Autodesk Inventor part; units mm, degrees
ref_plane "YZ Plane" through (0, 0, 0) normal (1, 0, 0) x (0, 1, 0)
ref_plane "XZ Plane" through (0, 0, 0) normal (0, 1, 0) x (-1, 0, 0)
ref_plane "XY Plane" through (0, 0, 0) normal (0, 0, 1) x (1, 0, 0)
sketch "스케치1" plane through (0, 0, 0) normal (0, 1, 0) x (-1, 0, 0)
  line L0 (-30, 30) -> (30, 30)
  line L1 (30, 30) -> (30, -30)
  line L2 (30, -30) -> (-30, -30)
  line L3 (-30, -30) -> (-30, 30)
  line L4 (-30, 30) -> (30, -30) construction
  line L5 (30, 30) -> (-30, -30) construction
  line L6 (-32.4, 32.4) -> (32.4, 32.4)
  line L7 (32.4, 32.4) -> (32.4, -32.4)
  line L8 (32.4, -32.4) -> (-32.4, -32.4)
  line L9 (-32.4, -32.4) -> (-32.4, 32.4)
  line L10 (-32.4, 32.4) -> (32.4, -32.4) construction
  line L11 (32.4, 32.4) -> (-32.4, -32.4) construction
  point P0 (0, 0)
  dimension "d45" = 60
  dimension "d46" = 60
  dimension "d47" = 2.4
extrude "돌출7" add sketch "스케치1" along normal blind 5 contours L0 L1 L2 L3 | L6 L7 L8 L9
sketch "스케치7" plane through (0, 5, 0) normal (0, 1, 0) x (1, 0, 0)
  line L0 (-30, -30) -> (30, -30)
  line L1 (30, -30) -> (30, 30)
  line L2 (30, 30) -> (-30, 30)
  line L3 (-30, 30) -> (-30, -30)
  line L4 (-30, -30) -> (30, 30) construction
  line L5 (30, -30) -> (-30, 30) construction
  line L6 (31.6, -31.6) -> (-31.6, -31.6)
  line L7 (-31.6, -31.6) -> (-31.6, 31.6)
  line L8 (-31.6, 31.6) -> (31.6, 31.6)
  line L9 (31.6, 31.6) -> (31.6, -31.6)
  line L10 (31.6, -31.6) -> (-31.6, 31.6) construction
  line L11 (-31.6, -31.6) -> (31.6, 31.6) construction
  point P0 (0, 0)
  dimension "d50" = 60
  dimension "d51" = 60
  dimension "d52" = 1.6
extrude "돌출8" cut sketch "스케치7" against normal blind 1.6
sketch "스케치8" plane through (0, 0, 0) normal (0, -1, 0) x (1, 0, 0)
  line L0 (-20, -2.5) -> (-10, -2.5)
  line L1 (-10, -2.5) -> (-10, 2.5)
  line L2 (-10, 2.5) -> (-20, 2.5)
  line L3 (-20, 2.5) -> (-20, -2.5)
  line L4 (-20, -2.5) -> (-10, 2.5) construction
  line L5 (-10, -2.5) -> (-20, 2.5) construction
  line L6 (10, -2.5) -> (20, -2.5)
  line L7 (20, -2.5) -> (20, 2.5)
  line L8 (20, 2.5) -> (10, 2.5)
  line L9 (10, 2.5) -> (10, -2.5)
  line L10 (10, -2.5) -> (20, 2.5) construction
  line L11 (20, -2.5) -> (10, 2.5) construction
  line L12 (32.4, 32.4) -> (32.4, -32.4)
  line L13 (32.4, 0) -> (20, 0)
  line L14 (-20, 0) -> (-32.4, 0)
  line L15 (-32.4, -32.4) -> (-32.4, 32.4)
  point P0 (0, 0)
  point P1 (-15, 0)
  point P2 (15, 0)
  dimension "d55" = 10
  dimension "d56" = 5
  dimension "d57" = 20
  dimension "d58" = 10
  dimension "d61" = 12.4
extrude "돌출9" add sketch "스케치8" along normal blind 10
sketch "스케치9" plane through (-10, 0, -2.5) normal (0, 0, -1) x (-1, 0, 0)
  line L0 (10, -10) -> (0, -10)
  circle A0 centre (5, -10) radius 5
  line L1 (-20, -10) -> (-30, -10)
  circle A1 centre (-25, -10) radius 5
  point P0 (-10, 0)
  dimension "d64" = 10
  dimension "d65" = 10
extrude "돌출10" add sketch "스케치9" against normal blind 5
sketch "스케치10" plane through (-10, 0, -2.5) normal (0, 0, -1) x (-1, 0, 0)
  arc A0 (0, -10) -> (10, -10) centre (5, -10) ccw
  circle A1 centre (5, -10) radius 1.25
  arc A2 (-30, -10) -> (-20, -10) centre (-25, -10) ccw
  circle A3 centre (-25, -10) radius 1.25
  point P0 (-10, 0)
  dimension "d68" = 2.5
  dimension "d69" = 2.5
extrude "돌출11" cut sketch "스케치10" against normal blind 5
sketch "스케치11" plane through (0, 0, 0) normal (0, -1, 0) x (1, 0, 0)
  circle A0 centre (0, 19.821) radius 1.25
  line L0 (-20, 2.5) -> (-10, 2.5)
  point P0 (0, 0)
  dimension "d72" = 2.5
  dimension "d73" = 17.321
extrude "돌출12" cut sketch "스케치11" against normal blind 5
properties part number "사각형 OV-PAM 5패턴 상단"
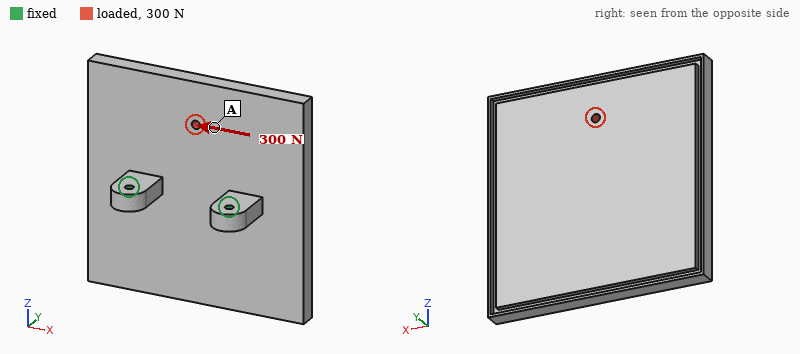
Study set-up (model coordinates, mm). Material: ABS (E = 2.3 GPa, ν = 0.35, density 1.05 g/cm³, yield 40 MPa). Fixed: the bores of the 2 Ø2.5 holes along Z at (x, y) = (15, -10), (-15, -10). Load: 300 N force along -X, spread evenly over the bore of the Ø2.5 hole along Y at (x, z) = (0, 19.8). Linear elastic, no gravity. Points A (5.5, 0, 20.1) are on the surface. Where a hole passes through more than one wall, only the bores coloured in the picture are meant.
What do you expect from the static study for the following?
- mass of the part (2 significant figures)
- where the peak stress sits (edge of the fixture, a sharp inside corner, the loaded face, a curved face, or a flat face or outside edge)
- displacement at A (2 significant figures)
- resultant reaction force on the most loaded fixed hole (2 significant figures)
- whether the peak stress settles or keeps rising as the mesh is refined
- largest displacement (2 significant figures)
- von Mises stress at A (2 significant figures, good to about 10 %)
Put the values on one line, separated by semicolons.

23 g; edge of the fixture; 0.46 mm; 240 N; keeps rising; 0.77 mm; 4.8 MPa
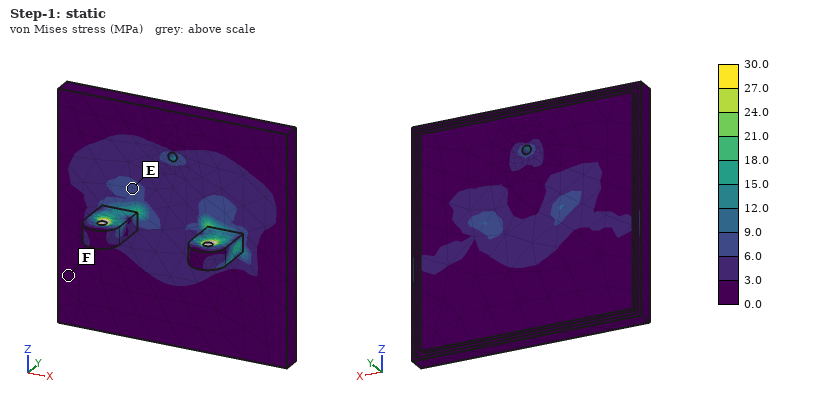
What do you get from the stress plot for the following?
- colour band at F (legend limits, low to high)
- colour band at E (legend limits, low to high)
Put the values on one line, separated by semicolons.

0.0 to 3.0 MPa; 6.0 to 9.0 MPa
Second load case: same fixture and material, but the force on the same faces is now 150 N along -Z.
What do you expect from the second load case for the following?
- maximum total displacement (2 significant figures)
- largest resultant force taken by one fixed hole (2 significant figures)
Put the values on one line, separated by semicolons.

0.88 mm; 75 N
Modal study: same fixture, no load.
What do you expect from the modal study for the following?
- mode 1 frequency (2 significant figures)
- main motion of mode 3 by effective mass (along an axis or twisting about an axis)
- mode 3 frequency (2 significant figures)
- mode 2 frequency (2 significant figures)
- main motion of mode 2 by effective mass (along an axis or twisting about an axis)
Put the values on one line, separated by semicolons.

340 Hz; along Y; 1200 Hz; 810 Hz; twisting about Y
